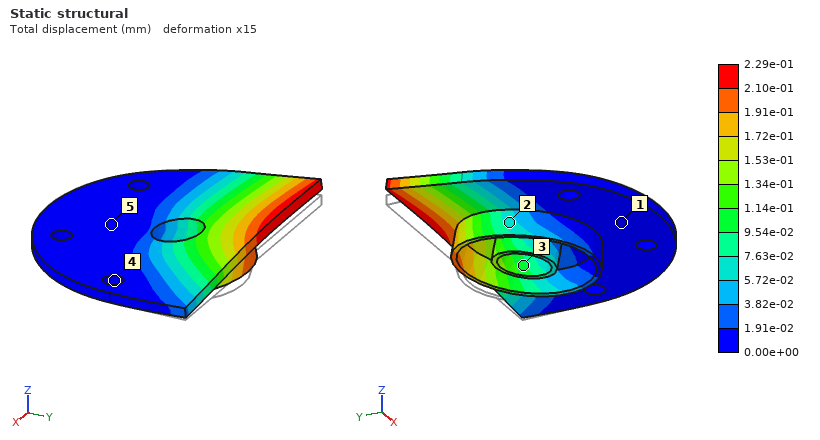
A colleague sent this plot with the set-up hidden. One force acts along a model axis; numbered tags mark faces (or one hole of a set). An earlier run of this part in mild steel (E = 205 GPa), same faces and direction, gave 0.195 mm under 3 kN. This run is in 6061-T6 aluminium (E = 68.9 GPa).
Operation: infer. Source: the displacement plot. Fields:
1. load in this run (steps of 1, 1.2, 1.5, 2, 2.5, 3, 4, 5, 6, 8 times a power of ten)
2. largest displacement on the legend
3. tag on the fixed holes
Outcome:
1.2 kN
2.29e-01 mm
4
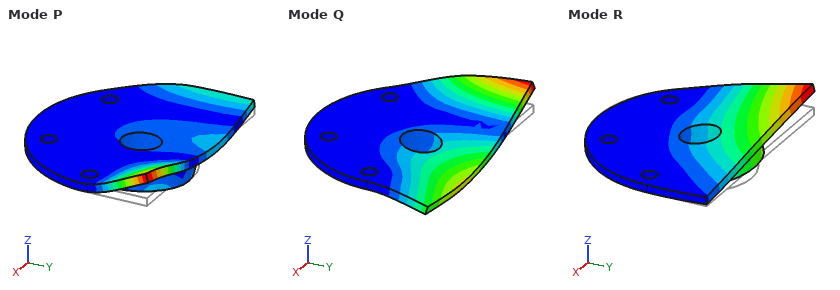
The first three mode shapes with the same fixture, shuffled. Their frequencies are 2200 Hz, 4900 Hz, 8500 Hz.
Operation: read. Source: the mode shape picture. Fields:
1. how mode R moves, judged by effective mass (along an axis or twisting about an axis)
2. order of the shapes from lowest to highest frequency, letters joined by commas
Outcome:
along Z
R, Q, P
